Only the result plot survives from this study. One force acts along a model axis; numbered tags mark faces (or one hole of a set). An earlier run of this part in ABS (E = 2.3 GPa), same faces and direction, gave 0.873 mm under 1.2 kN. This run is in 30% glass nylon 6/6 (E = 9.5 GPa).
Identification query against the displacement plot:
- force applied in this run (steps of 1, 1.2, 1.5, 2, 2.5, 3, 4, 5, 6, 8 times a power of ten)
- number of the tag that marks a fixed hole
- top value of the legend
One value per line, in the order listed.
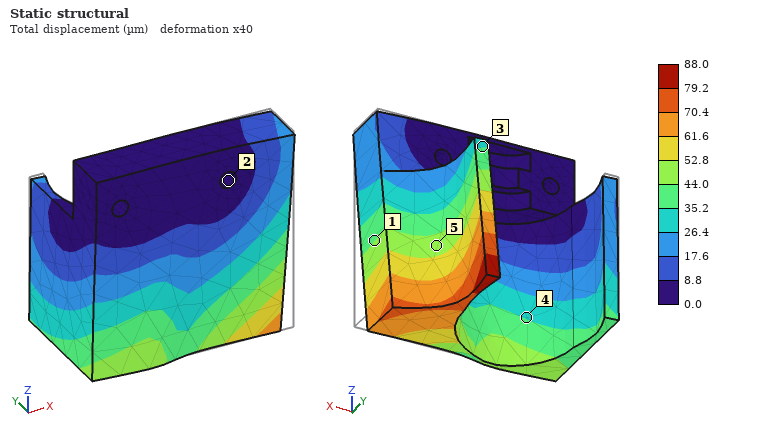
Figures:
500 N
2
88.0 µm
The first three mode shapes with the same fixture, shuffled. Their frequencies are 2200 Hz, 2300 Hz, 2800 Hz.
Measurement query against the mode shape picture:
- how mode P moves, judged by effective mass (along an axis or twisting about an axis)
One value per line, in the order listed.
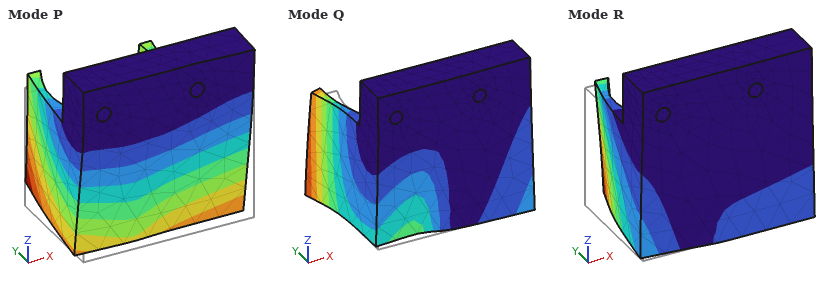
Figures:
along Y
